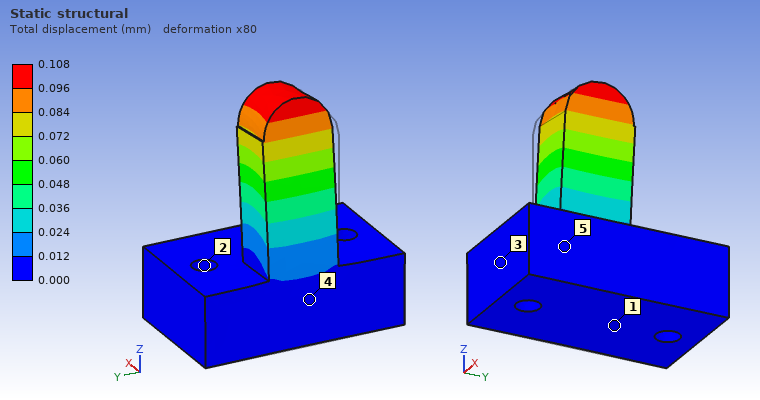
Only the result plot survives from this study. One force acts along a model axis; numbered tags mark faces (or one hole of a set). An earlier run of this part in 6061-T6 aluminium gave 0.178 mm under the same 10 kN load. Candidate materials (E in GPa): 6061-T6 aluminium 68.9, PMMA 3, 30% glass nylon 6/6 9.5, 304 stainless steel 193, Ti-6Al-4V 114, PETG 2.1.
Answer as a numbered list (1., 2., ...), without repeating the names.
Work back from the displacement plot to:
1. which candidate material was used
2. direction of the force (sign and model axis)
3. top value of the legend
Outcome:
1. Ti-6Al-4V
2. +X
3. 0.108 mm
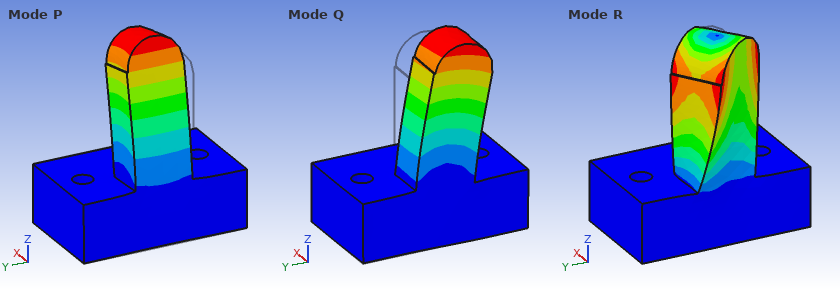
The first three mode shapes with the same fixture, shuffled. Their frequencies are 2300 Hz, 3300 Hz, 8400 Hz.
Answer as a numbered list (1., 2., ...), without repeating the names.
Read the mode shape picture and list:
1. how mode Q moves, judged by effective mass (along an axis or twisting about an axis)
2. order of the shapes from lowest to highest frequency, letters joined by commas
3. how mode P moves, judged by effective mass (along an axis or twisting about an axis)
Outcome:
1. along Y
2. P, Q, R
3. along X
